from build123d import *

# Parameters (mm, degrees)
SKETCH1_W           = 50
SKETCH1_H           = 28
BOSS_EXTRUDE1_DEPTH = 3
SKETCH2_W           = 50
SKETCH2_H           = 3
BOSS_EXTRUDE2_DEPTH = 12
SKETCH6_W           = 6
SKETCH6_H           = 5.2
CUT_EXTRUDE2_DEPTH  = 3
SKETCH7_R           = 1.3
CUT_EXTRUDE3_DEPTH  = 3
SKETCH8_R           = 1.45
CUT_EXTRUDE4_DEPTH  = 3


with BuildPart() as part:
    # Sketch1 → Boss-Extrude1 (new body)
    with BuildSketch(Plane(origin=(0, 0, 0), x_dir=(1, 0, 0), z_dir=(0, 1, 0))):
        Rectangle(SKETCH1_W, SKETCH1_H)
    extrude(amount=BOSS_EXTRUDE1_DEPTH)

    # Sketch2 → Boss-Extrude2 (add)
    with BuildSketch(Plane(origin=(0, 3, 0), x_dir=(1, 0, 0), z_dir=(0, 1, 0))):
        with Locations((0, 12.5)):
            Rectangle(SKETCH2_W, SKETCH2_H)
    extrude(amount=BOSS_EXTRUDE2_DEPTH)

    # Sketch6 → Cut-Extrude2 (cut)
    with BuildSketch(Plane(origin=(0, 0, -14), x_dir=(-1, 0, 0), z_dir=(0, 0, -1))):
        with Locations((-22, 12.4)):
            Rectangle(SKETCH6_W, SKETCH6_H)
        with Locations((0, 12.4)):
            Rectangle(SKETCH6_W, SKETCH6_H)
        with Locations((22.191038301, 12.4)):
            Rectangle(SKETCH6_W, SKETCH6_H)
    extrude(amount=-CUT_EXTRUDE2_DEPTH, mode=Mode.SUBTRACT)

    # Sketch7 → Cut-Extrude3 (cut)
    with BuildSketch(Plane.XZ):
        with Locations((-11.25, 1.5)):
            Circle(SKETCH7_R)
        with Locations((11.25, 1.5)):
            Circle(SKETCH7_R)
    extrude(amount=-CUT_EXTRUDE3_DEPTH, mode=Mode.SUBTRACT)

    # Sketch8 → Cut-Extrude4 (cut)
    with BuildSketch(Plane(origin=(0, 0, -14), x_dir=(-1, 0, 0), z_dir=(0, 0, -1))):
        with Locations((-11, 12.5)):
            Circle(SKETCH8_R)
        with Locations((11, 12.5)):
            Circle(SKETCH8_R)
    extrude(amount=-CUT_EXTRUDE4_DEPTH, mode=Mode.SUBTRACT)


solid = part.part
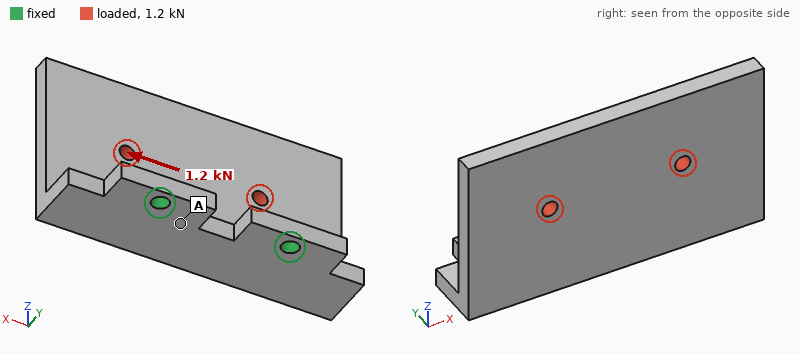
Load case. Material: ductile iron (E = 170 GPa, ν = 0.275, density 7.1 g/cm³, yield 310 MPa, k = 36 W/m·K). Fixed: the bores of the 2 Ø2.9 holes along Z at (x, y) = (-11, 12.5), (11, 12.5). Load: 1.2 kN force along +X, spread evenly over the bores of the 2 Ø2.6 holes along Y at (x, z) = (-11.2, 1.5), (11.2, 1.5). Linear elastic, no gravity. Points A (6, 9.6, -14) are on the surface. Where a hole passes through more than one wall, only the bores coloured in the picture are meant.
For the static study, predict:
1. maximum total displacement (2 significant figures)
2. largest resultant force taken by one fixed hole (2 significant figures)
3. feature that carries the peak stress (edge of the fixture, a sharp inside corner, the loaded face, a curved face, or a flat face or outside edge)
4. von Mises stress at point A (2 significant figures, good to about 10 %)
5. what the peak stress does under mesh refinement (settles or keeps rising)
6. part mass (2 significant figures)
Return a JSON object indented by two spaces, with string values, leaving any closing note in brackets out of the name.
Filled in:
{
  "maximum total displacement": "93 µm",
  "largest resultant force taken by one fixed hole": "1.0 kN",
  "feature that carries the peak stress": "edge of the fixture",
  "von Mises stress at point A": "35 MPa",
  "what the peak stress does under mesh refinement": "keeps rising",
  "part mass": "40 g"
}
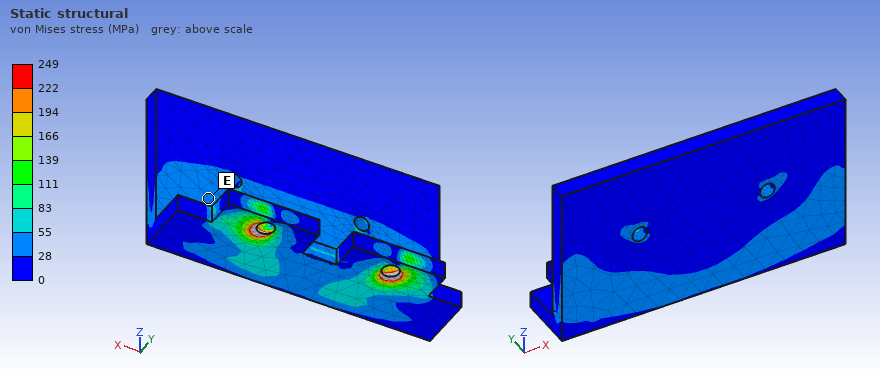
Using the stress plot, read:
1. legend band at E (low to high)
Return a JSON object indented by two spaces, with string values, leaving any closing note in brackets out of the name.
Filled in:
{
  "legend band at E": "28 to 55 MPa"
}
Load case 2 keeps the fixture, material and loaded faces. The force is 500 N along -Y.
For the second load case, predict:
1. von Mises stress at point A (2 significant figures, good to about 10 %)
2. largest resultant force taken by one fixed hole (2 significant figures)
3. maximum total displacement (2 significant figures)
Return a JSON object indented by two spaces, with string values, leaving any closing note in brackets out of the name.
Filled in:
{
  "von Mises stress at point A": "100 MPa",
  "largest resultant force taken by one fixed hole": "250 N",
  "maximum total displacement": "0.20 mm"
}
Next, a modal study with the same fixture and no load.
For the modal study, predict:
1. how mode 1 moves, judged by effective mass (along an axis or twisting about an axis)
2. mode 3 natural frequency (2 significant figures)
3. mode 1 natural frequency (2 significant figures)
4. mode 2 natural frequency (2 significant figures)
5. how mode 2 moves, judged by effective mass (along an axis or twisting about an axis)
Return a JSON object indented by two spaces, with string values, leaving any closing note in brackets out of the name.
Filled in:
{
  "how mode 1 moves, judged by effective mass": "along Y",
  "mode 3 natural frequency": "5200 Hz",
  "mode 1 natural frequency": "1800 Hz",
  "mode 2 natural frequency": "3300 Hz",
  "how mode 2 moves, judged by effective mass": "along X"
}
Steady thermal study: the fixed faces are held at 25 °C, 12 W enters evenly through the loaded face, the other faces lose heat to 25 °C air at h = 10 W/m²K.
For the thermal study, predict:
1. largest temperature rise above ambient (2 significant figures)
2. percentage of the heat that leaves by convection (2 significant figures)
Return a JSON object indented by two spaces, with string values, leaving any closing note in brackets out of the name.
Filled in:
{
  "largest temperature rise above ambient": "71 K",
  "percentage of the heat that leaves by convection": "15 %"
}
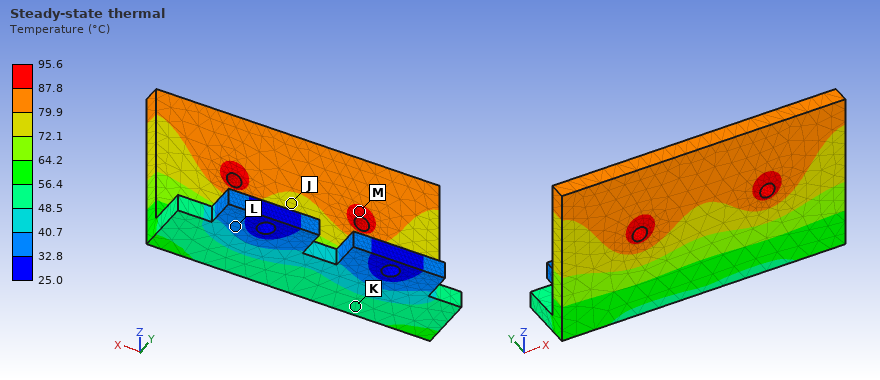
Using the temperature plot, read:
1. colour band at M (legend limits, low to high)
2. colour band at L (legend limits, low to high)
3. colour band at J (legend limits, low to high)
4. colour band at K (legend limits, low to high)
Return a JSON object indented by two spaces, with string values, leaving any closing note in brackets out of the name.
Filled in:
{
  "colour band at M": "87.8 to 95.6 °C",
  "colour band at L": "32.8 to 40.7 °C",
  "colour band at J": "72.1 to 79.9 °C",
  "colour band at K": "48.5 to 56.4 °C"
}
